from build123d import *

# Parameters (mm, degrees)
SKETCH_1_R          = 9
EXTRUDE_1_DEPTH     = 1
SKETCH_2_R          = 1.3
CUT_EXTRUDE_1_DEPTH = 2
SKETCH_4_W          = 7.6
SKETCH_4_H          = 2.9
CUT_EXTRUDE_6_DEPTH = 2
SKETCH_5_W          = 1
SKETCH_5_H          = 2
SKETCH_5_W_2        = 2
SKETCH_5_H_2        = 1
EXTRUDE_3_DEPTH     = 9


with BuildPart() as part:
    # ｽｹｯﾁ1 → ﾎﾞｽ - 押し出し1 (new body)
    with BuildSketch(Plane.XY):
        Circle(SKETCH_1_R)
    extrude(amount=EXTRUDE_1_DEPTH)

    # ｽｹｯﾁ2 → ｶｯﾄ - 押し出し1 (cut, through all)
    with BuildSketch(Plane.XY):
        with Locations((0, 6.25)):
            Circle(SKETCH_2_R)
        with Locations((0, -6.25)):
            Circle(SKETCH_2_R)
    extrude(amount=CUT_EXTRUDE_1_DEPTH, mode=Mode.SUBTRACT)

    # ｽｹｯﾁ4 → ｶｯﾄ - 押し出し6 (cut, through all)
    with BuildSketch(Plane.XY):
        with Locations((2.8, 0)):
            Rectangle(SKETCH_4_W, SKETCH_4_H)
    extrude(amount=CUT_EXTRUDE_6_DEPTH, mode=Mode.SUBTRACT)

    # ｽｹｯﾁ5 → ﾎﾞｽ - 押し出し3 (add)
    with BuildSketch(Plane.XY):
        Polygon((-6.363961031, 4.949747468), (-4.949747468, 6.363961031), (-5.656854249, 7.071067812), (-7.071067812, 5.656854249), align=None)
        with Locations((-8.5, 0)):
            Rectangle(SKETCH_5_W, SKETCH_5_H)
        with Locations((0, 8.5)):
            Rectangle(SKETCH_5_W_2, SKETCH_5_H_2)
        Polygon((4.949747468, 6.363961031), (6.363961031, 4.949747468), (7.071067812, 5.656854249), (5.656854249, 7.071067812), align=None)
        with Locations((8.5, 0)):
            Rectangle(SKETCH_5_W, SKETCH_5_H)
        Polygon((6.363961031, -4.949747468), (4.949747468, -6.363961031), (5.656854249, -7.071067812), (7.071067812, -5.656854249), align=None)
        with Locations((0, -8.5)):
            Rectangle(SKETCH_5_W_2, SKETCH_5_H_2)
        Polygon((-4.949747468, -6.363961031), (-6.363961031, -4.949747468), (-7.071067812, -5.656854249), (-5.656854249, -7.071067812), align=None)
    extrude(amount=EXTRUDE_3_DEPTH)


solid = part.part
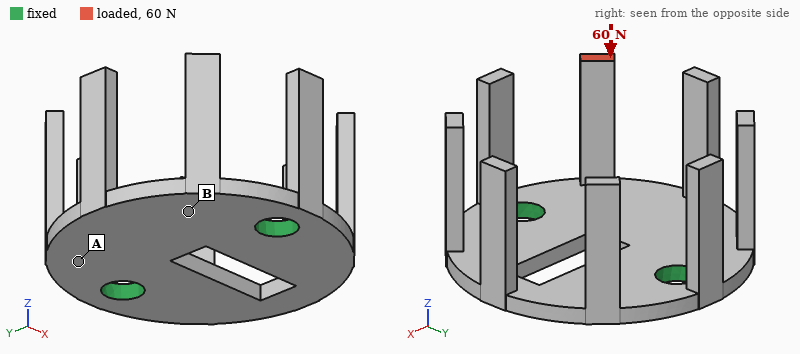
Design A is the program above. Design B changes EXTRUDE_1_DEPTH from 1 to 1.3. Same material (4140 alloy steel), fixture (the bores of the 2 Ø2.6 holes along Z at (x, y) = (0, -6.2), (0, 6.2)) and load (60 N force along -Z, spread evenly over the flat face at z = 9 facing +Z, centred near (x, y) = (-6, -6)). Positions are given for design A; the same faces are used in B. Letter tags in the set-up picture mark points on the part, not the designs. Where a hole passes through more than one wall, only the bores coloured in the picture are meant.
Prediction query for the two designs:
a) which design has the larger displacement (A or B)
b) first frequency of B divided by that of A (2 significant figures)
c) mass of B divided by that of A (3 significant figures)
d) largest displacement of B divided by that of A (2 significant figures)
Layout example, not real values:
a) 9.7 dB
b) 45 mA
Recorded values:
a) A
b) 1.3
c) 1.18
d) 0.48
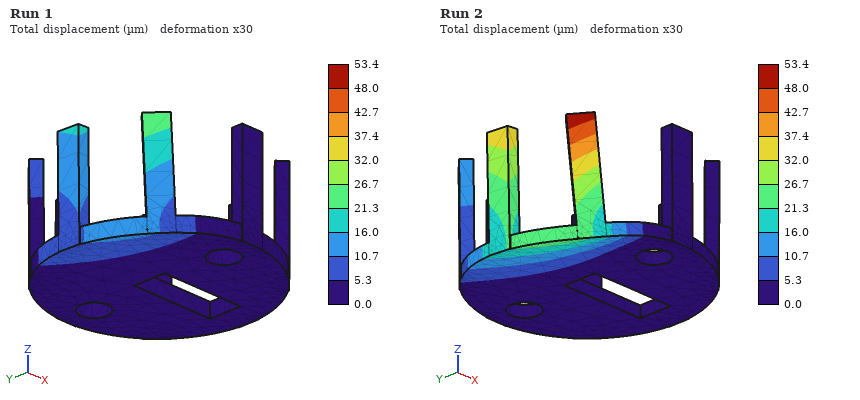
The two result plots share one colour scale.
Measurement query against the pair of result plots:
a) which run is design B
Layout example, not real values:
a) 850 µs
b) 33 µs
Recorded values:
a) Run 1
